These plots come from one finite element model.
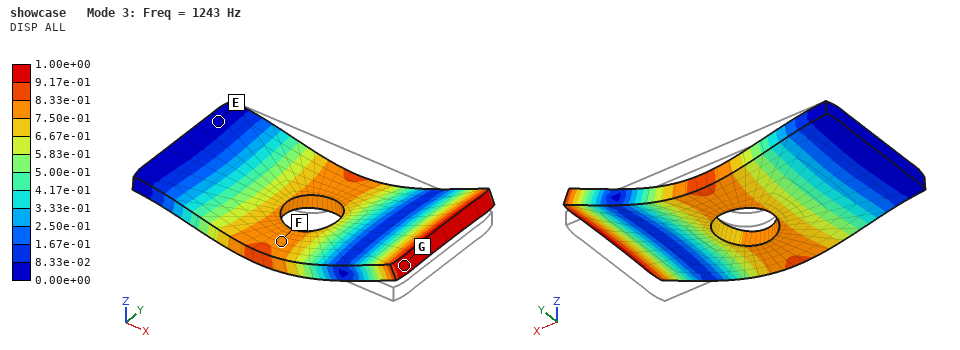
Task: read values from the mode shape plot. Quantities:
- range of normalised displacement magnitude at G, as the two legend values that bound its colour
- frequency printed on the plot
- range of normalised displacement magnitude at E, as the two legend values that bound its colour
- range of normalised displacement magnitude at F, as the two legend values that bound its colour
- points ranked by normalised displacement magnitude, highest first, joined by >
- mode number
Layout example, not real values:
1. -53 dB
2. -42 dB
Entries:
1. 9.17e-01 to 1.00e+00
2. 1243 Hz
3. 0.00e+00 to 8.33e-02
4. 7.50e-01 to 8.33e-01
5. G > F > E
6. 3
